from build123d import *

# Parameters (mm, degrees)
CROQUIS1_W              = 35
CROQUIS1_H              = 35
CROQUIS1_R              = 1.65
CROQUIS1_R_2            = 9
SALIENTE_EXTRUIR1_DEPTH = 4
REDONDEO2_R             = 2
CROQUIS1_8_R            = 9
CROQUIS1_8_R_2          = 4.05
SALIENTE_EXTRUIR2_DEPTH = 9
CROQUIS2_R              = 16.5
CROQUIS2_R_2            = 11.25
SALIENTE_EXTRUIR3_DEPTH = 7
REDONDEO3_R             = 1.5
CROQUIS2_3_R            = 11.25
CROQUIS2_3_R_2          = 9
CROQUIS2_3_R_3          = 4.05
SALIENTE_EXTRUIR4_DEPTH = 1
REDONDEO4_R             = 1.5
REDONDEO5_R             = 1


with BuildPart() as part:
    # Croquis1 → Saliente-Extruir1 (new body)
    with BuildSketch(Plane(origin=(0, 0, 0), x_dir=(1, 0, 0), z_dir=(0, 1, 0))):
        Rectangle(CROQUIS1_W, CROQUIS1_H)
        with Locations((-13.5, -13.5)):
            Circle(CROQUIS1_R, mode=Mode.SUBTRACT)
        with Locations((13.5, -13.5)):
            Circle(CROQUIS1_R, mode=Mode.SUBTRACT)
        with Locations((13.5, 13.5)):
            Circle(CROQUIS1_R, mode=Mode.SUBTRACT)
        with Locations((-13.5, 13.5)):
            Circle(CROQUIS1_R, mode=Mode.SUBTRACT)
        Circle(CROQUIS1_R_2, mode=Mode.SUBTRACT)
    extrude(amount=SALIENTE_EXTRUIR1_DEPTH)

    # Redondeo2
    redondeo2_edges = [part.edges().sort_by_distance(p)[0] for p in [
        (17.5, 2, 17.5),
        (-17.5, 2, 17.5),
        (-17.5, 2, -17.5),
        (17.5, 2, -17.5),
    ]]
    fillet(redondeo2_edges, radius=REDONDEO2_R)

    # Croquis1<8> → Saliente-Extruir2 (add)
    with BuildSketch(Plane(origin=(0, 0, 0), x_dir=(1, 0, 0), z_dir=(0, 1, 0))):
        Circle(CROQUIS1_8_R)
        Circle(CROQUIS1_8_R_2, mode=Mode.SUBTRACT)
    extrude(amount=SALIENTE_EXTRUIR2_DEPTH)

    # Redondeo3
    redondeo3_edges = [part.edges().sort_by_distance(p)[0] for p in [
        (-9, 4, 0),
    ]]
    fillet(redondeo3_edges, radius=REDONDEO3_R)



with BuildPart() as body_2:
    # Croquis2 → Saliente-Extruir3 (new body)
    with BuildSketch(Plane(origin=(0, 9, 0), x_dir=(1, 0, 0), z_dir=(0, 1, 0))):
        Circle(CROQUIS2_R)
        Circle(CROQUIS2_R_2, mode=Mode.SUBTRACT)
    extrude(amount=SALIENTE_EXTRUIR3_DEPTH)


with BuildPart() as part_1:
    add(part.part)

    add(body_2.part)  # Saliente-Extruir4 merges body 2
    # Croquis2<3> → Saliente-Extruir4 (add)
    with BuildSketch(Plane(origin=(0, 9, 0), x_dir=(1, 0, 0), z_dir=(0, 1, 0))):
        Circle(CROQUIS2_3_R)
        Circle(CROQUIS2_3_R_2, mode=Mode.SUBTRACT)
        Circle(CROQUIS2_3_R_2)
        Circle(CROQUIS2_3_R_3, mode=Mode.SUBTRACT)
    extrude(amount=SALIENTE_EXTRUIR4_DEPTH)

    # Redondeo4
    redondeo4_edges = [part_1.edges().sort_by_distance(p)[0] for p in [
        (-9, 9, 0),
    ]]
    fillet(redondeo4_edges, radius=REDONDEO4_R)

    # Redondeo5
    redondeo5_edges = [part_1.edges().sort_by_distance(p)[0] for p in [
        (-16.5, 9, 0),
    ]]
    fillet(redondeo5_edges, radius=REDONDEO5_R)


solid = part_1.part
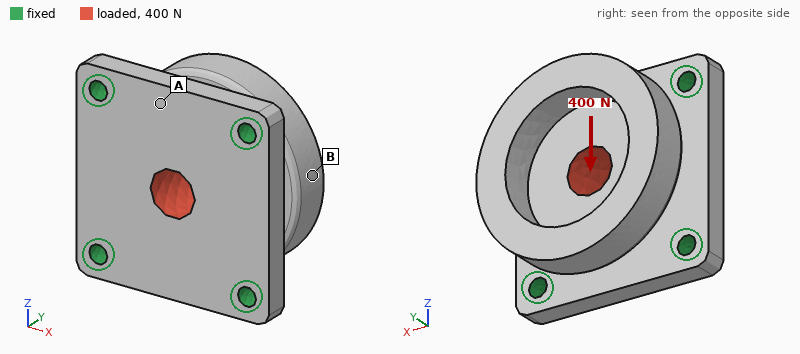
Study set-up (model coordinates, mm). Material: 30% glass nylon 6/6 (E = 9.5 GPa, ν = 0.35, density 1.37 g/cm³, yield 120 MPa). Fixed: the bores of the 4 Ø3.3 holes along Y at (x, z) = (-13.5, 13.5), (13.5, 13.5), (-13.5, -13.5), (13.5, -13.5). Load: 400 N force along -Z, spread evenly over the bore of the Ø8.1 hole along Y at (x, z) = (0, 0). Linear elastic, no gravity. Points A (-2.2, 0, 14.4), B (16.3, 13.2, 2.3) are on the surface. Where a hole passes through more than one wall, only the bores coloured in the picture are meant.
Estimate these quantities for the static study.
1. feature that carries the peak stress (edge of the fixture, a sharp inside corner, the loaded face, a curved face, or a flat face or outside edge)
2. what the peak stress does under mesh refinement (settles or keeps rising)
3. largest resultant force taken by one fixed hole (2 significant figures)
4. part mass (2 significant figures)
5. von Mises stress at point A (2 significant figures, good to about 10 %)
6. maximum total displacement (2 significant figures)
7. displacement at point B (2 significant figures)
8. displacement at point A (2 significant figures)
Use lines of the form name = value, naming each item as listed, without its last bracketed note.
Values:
feature that carries the peak stress = edge of the fixture
what the peak stress does under mesh refinement = keeps rising
largest resultant force taken by one fixed hole = 110 N
part mass = 13 g
von Mises stress at point A = 2.1 MPa
maximum total displacement = 14 µm
displacement at point B = 11 µm
displacement at point A = 6.2 µm
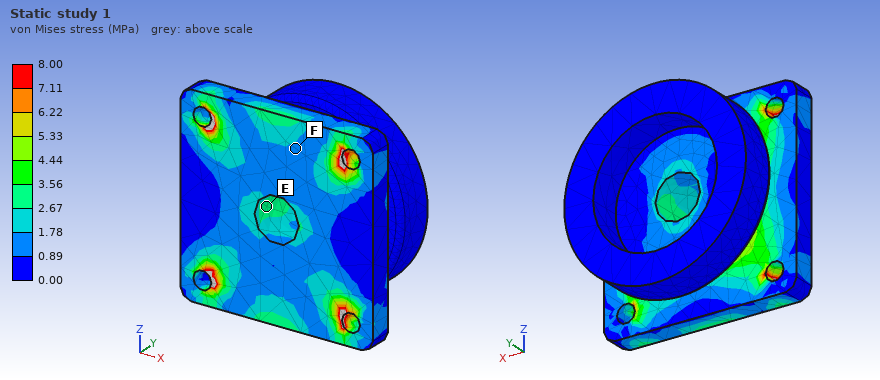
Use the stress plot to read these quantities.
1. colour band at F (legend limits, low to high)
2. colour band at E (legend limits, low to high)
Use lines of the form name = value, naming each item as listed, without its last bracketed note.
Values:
colour band at F = 0.89 to 1.78 MPa
colour band at E = 2.67 to 3.56 MPa
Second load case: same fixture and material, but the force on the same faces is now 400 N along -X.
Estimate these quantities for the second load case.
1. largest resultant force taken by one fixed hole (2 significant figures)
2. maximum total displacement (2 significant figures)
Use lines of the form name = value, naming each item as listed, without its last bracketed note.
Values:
largest resultant force taken by one fixed hole = 110 N
maximum total displacement = 14 µm
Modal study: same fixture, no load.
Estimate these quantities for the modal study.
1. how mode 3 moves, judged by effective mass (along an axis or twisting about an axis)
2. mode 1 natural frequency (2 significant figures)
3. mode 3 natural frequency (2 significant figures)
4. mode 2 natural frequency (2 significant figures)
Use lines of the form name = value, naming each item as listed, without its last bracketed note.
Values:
how mode 3 moves, judged by effective mass = along Y
mode 1 natural frequency = 4700 Hz
mode 3 natural frequency = 6200 Hz
mode 2 natural frequency = 4700 Hz
